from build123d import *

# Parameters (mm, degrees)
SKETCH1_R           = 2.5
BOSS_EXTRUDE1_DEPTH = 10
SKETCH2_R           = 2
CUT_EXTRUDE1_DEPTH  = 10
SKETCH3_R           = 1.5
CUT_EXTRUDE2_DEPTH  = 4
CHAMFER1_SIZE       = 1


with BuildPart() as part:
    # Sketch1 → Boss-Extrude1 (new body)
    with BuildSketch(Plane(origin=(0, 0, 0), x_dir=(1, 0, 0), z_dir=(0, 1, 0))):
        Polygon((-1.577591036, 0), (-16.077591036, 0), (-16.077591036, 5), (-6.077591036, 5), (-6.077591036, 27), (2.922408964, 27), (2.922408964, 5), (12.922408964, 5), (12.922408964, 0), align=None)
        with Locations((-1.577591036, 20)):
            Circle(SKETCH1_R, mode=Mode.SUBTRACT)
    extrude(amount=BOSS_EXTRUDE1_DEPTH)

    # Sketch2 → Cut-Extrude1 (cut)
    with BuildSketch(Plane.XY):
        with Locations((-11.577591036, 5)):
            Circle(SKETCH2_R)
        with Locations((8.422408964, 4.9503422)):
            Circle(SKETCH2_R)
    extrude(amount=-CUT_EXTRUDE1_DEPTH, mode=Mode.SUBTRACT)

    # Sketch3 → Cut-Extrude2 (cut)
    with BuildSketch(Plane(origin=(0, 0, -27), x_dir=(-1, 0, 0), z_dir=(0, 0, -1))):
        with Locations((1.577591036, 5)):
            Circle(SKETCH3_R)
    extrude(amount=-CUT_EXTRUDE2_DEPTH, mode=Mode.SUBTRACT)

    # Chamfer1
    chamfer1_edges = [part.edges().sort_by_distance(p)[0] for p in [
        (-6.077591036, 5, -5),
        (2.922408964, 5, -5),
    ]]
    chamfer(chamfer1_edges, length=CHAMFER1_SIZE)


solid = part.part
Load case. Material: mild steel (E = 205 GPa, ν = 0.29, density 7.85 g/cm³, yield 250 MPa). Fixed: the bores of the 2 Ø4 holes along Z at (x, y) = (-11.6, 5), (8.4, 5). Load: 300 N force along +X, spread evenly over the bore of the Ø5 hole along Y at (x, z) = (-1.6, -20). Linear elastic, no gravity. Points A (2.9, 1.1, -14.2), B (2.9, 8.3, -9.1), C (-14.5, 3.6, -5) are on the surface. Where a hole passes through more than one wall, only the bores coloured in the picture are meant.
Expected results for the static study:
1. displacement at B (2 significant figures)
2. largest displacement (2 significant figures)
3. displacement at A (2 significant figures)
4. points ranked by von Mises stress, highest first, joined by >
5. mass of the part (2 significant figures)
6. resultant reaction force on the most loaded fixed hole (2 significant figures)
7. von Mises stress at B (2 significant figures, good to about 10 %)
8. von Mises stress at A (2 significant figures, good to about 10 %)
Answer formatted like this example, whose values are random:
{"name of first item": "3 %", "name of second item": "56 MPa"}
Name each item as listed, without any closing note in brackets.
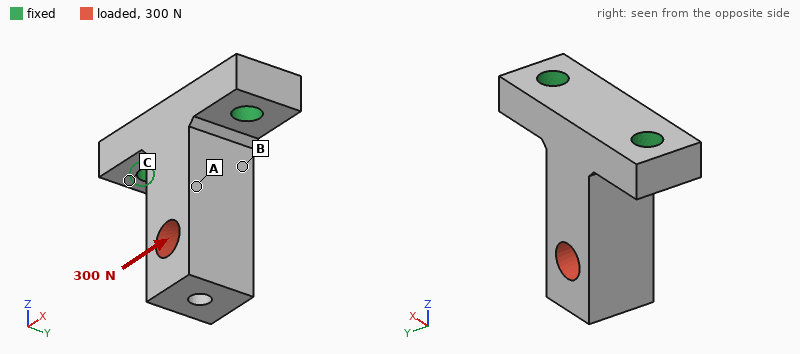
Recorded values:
{"displacement at B": "1.7 µm", "largest displacement": "9.4 µm", "displacement at A": "3.5 µm", "points ranked by von Mises stress, highest first, joined by >": "B > A > C", "mass of the part": "24 g", "resultant reaction force on the most loaded fixed hole": "380 N", "von Mises stress at B": "24 MPa", "von Mises stress at A": "14 MPa"}
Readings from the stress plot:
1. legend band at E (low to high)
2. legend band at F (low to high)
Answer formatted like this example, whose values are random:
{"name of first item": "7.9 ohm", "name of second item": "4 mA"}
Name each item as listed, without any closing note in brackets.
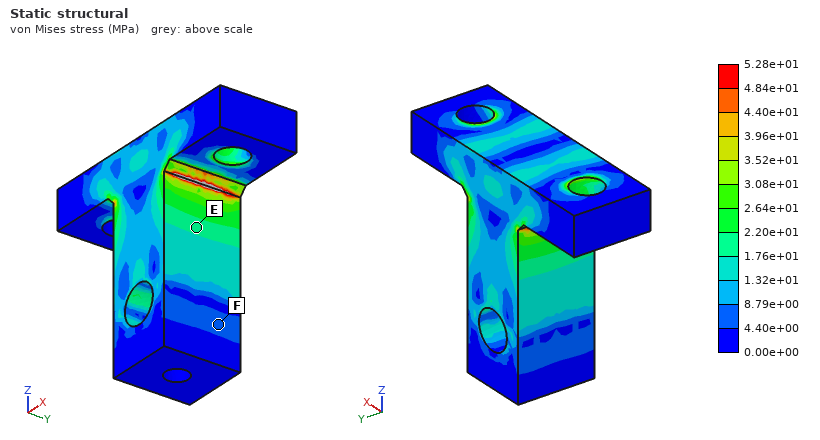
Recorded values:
{"legend band at E": "1.76e+01 to 2.20e+01 MPa", "legend band at F": "4.40e+00 to 8.79e+00 MPa"}
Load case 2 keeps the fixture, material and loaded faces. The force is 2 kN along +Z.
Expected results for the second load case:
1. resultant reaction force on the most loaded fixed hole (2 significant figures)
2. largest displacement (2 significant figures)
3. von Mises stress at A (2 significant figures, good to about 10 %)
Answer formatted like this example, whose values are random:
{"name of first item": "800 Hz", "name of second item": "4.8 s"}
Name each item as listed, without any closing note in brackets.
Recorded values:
{"resultant reaction force on the most loaded fixed hole": "1.0 kN", "largest displacement": "5.6 µm", "von Mises stress at A": "27 MPa"}
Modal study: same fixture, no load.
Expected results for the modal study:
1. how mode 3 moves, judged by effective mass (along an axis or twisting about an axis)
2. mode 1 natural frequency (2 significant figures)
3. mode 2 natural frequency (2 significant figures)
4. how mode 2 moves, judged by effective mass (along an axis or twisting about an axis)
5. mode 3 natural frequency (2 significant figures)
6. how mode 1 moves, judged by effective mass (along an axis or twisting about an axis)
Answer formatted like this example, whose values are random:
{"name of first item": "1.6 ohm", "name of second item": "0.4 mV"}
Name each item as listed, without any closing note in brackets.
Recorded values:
{"how mode 3 moves, judged by effective mass": "along Z", "mode 1 natural frequency": "7800 Hz", "mode 2 natural frequency": "11 kHz", "how mode 2 moves, judged by effective mass": "along X", "mode 3 natural frequency": "30 kHz", "how mode 1 moves, judged by effective mass": "along Y"}
